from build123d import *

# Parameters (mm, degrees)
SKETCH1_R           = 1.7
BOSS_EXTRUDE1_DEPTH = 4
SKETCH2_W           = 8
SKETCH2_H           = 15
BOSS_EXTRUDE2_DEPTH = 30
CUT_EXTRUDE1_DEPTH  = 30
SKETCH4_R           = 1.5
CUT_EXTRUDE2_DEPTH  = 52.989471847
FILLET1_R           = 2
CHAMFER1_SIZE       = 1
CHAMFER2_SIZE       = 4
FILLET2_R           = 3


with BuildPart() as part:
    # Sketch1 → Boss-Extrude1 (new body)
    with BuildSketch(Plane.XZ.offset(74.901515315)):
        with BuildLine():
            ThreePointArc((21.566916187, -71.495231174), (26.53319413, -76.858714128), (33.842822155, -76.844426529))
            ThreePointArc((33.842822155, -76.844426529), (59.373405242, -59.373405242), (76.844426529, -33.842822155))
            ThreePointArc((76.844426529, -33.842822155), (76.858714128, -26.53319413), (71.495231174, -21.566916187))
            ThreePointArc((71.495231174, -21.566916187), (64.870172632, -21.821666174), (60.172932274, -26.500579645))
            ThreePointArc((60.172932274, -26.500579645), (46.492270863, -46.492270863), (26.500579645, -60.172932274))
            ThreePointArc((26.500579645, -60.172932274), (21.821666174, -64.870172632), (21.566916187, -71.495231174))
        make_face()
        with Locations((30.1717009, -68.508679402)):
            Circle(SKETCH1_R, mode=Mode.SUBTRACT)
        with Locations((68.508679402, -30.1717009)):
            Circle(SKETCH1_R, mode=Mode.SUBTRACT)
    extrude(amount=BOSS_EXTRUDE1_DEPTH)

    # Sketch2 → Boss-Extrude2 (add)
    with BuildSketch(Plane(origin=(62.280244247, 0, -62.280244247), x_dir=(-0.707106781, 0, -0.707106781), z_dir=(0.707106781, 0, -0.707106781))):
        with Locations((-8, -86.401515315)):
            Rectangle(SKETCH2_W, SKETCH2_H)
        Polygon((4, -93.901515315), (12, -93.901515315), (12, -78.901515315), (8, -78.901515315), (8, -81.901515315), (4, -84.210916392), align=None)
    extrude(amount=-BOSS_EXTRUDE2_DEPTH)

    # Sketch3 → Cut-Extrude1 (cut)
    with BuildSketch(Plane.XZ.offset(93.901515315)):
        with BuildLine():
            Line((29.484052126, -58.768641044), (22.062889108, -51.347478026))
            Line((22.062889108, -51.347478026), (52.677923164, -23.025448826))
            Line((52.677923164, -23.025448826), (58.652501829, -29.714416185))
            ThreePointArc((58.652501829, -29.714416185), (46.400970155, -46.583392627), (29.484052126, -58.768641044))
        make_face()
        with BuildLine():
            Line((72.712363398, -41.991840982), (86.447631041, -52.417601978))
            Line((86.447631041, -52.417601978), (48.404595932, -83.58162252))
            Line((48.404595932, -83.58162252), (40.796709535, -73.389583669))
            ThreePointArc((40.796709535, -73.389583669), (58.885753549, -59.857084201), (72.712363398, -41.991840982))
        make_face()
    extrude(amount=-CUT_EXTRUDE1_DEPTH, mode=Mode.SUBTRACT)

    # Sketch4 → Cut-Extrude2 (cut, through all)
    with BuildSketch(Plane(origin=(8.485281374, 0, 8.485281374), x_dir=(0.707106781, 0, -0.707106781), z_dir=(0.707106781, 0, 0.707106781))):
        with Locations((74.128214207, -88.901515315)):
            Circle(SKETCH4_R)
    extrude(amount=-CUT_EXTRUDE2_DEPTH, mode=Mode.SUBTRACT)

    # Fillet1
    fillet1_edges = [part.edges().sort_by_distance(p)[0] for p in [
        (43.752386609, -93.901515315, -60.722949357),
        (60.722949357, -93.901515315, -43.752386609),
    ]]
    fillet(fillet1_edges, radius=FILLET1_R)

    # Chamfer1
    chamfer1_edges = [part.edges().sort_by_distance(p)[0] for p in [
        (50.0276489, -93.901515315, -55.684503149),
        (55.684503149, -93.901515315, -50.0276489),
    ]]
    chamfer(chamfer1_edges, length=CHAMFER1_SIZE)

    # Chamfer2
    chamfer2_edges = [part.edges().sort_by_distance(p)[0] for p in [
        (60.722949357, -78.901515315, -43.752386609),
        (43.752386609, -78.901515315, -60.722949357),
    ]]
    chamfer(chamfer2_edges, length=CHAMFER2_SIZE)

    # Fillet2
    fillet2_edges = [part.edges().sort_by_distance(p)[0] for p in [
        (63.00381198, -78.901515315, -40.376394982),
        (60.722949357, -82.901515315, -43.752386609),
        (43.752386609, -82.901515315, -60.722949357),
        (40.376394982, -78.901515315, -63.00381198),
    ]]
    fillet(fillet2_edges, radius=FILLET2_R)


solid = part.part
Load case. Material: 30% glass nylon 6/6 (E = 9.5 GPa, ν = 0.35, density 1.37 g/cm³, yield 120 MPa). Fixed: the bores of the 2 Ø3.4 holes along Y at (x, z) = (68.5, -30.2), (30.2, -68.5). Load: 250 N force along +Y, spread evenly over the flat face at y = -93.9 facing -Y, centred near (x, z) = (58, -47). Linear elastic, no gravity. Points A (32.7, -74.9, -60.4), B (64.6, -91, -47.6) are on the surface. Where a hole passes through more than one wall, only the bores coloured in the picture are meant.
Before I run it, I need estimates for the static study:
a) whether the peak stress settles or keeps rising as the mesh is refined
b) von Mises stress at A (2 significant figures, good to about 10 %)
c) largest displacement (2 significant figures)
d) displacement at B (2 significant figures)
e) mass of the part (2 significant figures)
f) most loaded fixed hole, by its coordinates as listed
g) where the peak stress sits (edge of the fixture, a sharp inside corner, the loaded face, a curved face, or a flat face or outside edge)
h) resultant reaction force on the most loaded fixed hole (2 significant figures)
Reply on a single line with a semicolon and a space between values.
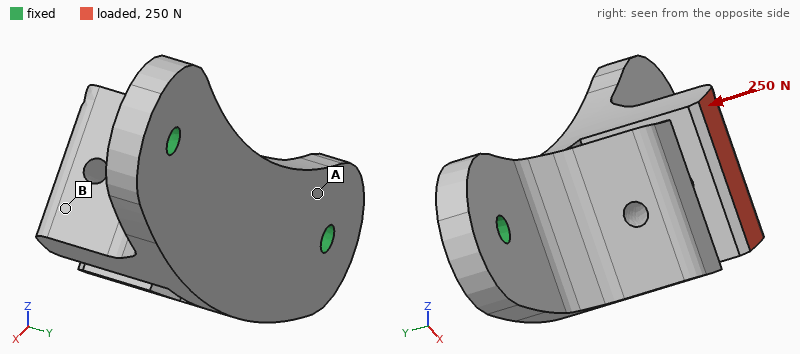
keeps rising; 13 MPa; 0.28 mm; 0.20 mm; 13 g; (68.5, -30.2); edge of the fixture; 170 N
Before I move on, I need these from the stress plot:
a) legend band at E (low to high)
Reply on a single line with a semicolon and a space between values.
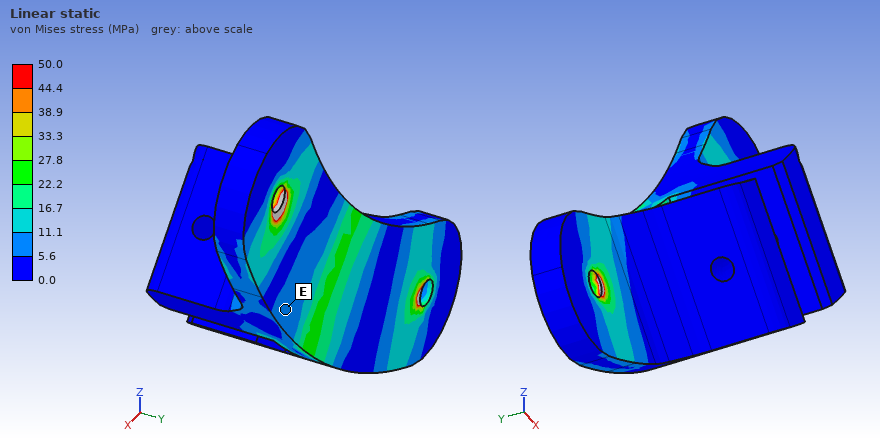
5.6 to 11.1 MPa
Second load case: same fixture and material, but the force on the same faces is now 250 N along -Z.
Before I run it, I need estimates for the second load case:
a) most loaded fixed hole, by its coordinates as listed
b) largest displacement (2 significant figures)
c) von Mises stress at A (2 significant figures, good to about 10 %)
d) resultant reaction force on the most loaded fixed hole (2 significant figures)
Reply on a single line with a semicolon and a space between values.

(68.5, -30.2); 0.50 mm; 18 MPa; 250 N
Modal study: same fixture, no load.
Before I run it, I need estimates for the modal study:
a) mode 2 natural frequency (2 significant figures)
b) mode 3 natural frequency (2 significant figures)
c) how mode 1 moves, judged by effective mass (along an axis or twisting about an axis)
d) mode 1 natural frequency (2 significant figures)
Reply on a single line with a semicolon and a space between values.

2500 Hz; 4400 Hz; along Y; 1800 Hz
